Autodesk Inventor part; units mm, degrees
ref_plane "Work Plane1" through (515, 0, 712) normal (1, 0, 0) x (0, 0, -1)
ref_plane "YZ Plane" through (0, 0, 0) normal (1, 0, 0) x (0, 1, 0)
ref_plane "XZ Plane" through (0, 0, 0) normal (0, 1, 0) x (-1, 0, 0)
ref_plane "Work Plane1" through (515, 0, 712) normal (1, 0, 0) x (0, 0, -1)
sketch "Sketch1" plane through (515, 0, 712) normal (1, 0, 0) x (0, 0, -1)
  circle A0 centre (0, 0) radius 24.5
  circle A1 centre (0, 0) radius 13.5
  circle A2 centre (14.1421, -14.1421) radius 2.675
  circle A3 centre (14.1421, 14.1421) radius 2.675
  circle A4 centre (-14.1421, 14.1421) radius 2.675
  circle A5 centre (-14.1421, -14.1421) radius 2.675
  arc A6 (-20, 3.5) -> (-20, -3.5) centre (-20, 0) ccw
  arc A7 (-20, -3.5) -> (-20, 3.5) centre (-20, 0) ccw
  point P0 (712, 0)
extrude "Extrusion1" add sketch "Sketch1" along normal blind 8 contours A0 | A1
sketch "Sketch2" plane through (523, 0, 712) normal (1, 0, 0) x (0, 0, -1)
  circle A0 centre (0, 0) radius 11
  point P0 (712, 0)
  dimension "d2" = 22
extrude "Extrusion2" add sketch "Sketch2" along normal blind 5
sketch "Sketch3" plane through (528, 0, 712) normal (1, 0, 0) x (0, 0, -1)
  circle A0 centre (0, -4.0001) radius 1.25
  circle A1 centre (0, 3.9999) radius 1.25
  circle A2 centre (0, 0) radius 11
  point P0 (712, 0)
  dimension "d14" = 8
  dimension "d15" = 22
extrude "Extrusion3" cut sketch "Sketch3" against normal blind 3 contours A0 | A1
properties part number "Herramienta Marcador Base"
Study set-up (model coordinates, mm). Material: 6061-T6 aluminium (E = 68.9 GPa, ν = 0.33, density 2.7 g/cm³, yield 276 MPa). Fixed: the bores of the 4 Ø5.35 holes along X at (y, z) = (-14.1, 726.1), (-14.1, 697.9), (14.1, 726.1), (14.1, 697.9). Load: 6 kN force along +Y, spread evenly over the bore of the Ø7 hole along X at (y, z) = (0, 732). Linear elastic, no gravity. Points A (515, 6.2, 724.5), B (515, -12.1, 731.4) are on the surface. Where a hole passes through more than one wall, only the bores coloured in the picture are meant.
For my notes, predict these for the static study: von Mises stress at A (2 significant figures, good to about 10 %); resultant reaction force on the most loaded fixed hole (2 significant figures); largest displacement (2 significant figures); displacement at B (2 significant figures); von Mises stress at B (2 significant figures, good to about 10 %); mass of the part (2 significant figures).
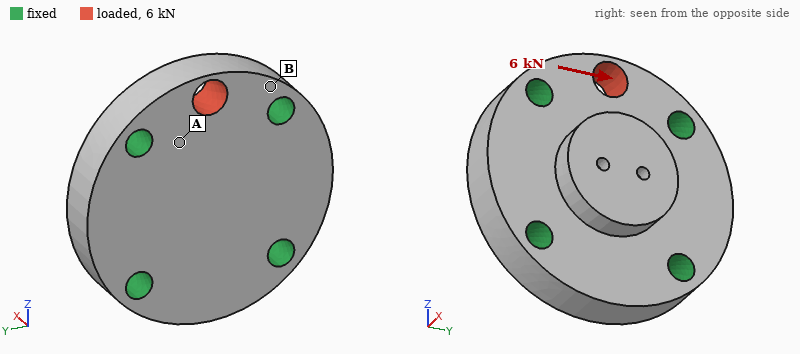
18 MPa
3.1 kN
16 µm
3.5 µm
40 MPa
43 g
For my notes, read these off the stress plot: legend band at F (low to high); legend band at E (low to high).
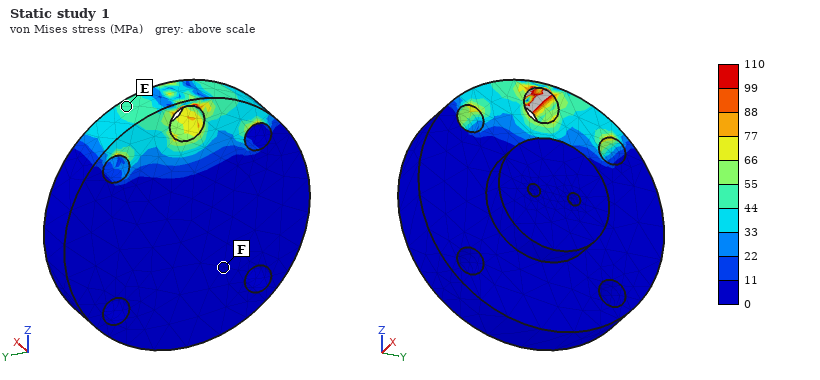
0 to 11 MPa
44 to 55 MPa
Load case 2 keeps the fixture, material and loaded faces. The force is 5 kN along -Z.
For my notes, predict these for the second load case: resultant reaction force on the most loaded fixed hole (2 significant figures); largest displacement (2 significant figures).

1.8 kN
22 µm
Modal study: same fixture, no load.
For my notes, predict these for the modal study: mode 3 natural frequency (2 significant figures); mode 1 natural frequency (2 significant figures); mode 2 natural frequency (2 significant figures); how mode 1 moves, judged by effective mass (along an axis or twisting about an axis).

35 kHz
29 kHz
35 kHz
along X
